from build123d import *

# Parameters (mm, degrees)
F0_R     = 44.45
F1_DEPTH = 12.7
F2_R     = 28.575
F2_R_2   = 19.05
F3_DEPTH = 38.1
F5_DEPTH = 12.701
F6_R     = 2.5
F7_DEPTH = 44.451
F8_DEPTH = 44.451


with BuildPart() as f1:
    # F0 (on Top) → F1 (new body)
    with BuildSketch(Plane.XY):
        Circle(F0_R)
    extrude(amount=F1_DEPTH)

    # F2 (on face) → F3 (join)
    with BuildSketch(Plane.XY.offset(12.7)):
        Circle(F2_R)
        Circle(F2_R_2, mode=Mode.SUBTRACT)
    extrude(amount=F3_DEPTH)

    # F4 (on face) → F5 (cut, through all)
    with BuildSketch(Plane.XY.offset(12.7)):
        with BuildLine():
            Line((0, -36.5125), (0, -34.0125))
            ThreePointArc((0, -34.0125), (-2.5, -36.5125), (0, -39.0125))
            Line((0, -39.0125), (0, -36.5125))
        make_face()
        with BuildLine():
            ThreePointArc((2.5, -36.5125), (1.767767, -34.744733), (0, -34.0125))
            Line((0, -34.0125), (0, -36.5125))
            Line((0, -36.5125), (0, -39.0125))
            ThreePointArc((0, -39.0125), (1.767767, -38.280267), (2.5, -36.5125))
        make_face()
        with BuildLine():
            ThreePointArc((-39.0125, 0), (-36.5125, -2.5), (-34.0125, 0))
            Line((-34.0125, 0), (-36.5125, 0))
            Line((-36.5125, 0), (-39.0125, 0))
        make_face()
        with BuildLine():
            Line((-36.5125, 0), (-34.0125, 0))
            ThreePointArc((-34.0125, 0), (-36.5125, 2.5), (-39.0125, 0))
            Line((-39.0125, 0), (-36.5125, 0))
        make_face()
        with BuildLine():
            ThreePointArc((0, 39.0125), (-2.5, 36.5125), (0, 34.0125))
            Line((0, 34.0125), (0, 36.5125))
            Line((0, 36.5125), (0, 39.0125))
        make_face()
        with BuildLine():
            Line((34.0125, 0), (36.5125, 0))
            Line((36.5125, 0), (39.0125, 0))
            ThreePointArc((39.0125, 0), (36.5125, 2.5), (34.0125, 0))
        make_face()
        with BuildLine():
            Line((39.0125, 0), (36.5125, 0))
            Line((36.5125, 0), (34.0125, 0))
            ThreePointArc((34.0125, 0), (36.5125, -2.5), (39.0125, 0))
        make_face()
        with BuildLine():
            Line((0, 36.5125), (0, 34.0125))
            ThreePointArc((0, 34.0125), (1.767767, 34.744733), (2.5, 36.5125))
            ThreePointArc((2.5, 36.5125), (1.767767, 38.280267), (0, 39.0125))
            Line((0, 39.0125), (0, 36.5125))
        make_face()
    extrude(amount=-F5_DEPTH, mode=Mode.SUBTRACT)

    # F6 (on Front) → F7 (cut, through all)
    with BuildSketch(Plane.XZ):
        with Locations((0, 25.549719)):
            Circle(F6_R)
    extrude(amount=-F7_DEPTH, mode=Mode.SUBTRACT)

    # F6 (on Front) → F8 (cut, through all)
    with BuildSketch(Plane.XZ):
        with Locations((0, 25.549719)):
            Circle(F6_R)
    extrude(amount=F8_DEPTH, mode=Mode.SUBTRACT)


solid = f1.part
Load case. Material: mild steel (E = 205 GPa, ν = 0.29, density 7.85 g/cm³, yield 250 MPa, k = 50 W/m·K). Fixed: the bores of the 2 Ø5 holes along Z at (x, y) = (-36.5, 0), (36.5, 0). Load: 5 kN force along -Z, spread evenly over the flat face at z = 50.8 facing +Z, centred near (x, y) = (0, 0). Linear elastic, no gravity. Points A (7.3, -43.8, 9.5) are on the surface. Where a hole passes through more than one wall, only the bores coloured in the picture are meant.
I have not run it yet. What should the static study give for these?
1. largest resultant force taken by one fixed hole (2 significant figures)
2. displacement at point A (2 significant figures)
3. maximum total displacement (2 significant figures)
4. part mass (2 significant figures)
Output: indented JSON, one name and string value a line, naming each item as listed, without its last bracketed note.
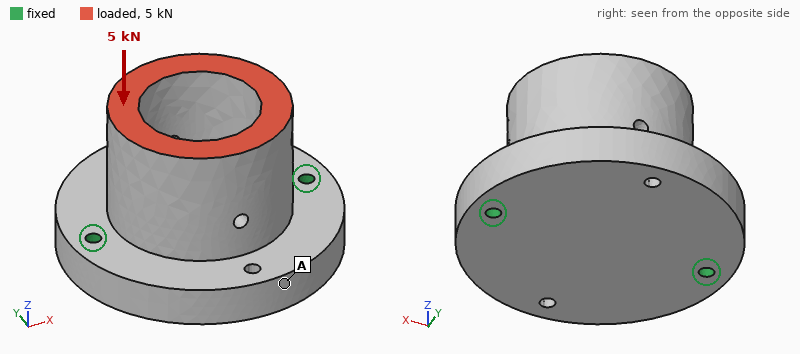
{
  "largest resultant force taken by one fixed hole": "2.6 kN",
  "displacement at point A": "4.5 µm",
  "maximum total displacement": "4.6 µm",
  "part mass": "1.0 kg"
}
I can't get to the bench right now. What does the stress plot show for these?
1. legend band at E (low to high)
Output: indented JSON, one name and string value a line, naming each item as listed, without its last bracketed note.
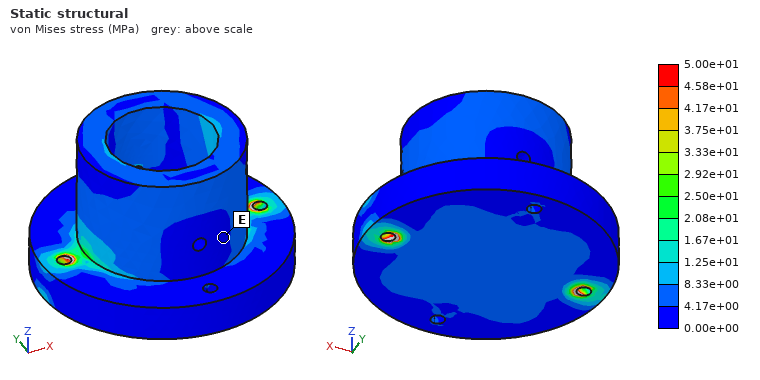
{
  "legend band at E": "0.00e+00 to 4.17e+00 MPa"
}
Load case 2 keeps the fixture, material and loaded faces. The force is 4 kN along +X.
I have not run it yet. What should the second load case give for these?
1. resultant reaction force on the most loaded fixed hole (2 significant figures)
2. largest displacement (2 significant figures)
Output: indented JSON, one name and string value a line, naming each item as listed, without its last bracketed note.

{
  "resultant reaction force on the most loaded fixed hole": "3.3 kN",
  "largest displacement": "8.8 µm"
}
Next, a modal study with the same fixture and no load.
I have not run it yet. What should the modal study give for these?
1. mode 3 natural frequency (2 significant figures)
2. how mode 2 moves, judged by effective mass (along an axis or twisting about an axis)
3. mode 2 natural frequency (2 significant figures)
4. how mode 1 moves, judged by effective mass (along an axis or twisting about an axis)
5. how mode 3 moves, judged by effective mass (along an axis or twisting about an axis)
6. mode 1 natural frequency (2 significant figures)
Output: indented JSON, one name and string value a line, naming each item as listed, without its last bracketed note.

{
  "mode 3 natural frequency": "8100 Hz",
  "how mode 2 moves, judged by effective mass": "along Z",
  "mode 2 natural frequency": "6000 Hz",
  "how mode 1 moves, judged by effective mass": "along Y",
  "how mode 3 moves, judged by effective mass": "along X",
  "mode 1 natural frequency": "2500 Hz"
}
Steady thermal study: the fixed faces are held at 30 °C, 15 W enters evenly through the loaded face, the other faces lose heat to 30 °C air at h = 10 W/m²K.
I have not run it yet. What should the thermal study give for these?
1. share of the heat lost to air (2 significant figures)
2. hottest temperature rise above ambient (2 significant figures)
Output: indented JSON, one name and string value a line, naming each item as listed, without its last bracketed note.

{
  "share of the heat lost to air": "12 %",
  "hottest temperature rise above ambient": "14 K"
}
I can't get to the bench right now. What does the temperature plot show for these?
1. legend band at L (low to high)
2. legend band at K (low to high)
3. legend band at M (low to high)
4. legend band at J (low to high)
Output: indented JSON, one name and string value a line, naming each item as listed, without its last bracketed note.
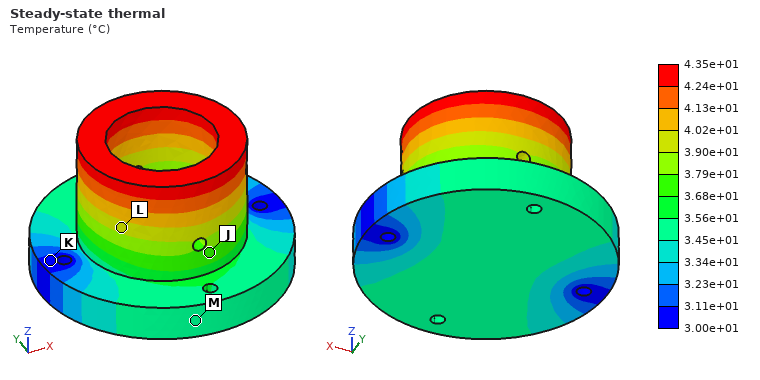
{
  "legend band at L": "3.90e+01 to 4.02e+01 °C",
  "legend band at K": "3.00e+01 to 3.11e+01 °C",
  "legend band at M": "3.45e+01 to 3.56e+01 °C",
  "legend band at J": "3.68e+01 to 3.79e+01 °C"
}
